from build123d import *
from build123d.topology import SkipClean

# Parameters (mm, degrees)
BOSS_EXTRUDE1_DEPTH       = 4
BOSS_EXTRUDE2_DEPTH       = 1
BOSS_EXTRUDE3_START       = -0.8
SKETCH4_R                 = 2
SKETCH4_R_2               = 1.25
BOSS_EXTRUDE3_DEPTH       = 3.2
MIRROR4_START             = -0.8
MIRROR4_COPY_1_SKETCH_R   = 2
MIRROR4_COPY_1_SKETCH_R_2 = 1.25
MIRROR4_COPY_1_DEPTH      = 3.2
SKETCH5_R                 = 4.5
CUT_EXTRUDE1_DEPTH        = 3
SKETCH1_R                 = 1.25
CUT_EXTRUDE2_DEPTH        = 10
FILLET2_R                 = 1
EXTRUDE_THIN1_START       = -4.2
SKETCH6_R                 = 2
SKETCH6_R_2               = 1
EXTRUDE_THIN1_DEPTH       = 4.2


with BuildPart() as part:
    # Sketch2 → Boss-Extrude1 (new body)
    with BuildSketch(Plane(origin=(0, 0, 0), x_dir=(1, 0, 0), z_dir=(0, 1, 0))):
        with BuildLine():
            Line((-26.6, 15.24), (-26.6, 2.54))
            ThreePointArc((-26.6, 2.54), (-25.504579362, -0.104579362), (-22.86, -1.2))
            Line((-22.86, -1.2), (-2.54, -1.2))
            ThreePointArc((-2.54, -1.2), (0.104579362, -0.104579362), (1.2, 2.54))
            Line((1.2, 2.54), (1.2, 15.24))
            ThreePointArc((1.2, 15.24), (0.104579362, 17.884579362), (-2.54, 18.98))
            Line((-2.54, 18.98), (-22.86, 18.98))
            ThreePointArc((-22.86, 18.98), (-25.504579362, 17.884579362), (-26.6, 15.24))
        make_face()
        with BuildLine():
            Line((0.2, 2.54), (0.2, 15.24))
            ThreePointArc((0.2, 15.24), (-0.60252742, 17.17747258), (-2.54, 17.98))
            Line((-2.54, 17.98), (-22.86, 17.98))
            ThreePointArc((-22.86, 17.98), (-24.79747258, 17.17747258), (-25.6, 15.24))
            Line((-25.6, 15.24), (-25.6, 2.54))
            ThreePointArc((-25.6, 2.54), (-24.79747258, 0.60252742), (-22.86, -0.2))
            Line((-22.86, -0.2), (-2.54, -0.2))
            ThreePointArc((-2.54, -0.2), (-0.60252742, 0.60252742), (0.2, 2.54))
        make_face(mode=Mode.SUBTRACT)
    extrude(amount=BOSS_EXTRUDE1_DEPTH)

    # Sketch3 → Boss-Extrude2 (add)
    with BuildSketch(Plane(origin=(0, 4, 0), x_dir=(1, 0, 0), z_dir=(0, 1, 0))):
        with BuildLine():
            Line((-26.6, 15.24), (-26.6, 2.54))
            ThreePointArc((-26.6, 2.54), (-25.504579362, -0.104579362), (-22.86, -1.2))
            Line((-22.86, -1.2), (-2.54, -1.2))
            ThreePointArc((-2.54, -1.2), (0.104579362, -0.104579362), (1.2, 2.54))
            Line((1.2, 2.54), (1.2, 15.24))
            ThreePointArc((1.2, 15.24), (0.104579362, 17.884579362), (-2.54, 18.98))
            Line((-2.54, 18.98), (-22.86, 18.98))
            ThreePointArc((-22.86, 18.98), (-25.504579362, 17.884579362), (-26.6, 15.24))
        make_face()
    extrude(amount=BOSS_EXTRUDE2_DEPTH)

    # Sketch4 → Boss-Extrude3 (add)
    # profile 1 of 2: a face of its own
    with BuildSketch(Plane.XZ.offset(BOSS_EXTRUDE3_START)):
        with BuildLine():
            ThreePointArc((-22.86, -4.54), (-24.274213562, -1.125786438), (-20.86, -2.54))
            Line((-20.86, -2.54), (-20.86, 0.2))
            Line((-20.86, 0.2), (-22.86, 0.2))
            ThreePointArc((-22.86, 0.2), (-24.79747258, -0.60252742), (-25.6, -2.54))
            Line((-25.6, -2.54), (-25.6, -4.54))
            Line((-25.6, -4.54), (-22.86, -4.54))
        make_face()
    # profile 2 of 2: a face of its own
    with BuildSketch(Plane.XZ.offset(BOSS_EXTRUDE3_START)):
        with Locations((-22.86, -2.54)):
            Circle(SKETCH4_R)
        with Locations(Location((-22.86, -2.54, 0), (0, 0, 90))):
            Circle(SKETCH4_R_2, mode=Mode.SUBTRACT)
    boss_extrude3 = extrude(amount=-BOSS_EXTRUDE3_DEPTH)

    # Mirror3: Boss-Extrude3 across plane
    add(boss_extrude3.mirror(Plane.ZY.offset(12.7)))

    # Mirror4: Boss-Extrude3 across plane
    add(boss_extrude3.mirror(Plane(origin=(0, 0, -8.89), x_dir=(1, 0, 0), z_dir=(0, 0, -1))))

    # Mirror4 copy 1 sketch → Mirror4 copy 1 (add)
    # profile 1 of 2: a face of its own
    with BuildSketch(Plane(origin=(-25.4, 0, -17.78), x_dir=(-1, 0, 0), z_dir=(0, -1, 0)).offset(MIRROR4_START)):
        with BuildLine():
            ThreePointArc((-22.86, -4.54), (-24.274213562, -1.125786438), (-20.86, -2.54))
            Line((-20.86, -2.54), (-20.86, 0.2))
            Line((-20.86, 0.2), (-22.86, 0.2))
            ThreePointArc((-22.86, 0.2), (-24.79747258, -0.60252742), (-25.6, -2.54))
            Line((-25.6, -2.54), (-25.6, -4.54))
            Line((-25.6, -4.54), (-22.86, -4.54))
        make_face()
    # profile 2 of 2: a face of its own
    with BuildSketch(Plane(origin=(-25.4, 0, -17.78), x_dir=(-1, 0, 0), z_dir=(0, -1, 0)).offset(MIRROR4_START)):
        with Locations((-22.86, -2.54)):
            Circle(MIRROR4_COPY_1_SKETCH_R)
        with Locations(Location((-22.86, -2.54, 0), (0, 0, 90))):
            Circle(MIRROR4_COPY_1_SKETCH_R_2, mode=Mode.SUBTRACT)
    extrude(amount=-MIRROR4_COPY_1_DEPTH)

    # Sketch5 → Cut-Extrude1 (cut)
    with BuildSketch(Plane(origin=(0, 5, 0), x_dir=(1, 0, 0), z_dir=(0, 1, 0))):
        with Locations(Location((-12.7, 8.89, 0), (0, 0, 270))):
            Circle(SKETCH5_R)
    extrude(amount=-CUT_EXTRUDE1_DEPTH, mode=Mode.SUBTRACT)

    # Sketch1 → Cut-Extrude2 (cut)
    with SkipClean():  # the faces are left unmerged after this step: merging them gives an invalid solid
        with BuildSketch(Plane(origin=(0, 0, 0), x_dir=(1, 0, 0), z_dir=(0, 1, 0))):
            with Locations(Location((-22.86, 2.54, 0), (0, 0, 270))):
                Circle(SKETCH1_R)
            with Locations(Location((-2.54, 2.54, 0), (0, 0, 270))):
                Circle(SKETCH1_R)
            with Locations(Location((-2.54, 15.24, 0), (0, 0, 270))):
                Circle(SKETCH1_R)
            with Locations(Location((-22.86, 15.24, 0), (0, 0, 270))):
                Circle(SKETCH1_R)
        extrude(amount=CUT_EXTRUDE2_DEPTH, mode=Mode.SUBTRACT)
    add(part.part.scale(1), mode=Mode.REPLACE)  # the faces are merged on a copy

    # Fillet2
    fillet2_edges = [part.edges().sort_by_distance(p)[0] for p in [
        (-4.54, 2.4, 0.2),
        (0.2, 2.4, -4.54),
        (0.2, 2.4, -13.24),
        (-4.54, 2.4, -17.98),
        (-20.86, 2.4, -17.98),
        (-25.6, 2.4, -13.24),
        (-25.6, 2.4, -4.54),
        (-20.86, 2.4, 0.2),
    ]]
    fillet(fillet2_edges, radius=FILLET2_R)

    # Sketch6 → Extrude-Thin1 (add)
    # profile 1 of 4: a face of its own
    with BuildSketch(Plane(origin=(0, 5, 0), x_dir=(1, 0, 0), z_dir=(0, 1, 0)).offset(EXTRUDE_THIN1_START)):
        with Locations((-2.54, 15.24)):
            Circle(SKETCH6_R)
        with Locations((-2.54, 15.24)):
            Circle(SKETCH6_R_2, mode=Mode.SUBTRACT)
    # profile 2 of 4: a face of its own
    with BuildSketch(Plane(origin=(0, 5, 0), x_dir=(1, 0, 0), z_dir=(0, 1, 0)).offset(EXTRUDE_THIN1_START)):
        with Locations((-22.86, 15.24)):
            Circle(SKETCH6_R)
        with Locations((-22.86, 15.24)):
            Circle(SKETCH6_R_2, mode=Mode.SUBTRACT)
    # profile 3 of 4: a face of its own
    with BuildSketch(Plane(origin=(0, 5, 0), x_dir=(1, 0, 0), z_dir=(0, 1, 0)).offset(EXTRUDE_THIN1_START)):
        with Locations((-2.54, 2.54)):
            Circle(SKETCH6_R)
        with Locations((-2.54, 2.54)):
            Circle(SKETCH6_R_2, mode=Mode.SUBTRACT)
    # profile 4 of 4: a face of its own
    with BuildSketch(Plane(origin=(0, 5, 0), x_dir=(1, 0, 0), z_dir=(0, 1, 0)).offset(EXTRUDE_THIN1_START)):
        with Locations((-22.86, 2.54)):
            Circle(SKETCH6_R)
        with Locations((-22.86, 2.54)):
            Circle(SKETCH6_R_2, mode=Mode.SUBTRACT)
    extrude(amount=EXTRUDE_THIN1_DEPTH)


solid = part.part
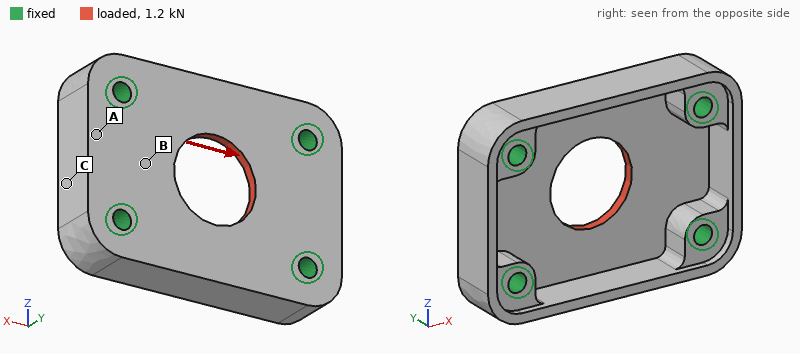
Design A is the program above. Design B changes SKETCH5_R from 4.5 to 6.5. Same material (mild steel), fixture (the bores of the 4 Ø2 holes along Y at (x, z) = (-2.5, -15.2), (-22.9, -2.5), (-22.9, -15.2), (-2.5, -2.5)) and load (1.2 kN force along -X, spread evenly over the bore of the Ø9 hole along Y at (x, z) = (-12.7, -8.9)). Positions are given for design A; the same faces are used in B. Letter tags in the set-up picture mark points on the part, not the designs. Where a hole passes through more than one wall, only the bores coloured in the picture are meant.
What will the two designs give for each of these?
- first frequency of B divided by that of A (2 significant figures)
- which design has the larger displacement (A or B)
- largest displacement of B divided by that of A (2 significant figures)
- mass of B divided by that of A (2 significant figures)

1.3
A
0.79
0.93
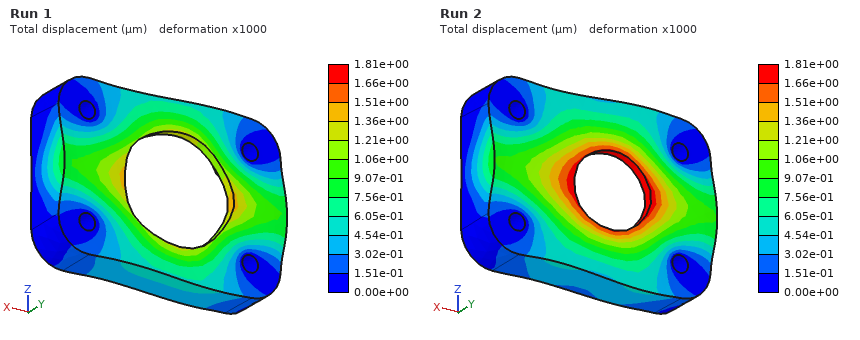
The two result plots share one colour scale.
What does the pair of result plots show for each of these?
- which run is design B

Run 1
